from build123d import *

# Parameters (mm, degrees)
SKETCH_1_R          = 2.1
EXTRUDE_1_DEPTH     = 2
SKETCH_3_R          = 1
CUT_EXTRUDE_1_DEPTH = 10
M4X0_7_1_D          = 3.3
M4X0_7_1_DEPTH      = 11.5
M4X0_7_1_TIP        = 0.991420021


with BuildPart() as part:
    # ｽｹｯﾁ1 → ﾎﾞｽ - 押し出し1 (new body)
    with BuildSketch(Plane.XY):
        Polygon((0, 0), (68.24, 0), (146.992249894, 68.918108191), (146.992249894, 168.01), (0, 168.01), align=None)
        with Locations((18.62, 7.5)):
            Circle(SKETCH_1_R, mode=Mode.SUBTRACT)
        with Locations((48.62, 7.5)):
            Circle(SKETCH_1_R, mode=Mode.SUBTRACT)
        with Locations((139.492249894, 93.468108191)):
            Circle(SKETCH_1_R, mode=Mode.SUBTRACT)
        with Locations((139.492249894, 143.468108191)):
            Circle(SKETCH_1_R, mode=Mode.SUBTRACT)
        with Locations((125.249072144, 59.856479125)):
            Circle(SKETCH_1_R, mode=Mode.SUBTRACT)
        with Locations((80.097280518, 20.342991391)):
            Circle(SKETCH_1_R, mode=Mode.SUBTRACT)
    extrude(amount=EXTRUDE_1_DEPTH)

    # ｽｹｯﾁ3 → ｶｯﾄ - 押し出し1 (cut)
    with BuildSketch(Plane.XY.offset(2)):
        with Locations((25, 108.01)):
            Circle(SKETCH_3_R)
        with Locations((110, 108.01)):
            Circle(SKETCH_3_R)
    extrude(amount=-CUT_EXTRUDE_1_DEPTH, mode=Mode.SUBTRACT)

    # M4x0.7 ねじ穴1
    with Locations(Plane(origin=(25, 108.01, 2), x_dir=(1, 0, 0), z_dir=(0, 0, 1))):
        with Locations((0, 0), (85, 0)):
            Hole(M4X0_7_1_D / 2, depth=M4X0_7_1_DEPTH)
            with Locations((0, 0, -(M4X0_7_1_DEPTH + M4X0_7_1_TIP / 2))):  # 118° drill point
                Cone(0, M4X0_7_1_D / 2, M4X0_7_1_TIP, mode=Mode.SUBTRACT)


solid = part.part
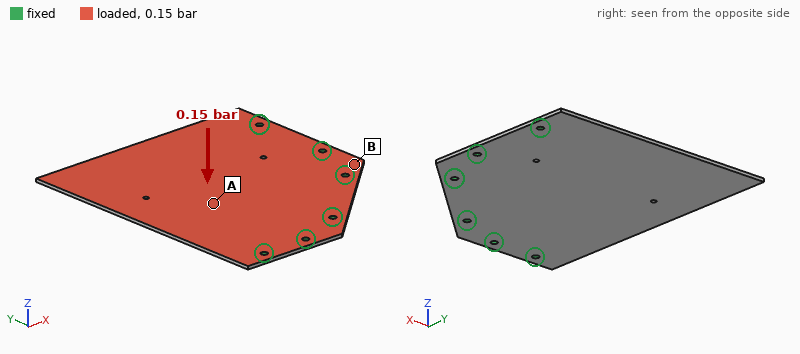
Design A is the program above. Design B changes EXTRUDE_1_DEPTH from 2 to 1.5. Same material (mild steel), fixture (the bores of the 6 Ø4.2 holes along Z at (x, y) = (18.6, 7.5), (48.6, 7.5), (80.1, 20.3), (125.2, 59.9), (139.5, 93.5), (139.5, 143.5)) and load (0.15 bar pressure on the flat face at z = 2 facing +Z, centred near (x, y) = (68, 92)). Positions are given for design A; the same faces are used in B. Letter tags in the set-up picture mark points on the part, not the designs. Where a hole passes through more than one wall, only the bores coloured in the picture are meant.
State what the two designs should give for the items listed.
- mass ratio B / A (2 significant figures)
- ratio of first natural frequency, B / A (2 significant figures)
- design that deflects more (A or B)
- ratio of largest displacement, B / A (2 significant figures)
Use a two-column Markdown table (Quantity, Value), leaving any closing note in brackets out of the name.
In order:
| Quantity | Value |
|---|---|
| mass ratio B / A | 0.75 |
| ratio of first natural frequency, B / A | 0.75 |
| design that deflects more | B |
| ratio of largest displacement, B / A | 2.4 |
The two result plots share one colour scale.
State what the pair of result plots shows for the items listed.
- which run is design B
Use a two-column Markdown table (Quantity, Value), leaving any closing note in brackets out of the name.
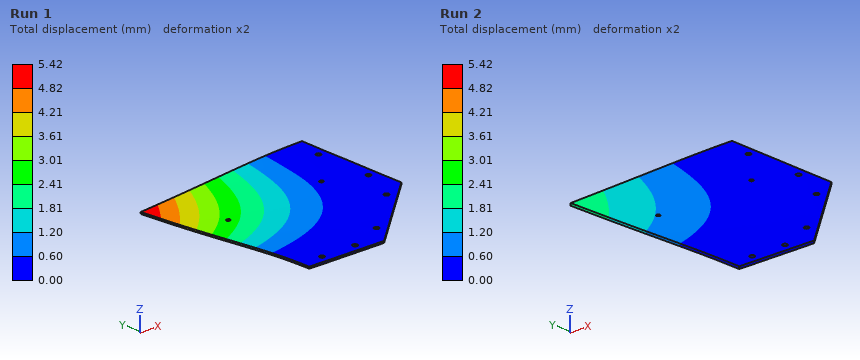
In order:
| Quantity | Value |
|---|---|
| which run is design B | Run 1 |
